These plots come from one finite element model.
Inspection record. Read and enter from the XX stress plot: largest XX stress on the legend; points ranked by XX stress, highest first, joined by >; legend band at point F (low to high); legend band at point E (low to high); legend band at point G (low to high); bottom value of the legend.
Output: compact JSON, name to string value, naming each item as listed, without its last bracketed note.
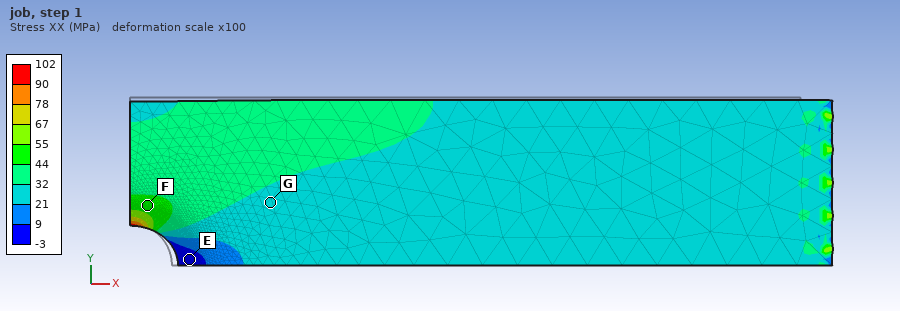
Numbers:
{"largest XX stress on the legend": "102 MPa", "points ranked by XX stress, highest first, joined by >": "F > G > E", "legend band at point F": "44 to 55 MPa", "legend band at point E": "-3 to 9 MPa", "legend band at point G": "21 to 32 MPa", "bottom value of the legend": "-3 MPa"}
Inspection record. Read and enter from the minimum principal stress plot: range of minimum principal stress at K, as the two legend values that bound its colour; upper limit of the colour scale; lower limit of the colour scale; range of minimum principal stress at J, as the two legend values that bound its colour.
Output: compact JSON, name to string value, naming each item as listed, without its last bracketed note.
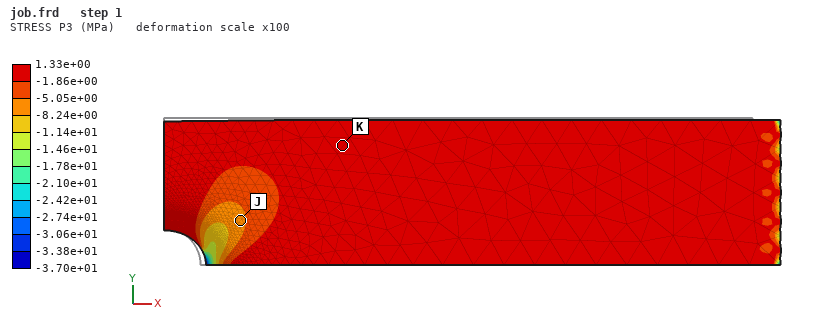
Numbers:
{"range of minimum principal stress at K, as the two legend values that bound its colour": "-1.86e+00 to 1.33e+00 MPa", "upper limit of the colour scale": "1.33e+00 MPa", "lower limit of the colour scale": "-3.70e+01 MPa", "range of minimum principal stress at J, as the two legend values that bound its colour": "-8.24e+00 to -5.05e+00 MPa"}
